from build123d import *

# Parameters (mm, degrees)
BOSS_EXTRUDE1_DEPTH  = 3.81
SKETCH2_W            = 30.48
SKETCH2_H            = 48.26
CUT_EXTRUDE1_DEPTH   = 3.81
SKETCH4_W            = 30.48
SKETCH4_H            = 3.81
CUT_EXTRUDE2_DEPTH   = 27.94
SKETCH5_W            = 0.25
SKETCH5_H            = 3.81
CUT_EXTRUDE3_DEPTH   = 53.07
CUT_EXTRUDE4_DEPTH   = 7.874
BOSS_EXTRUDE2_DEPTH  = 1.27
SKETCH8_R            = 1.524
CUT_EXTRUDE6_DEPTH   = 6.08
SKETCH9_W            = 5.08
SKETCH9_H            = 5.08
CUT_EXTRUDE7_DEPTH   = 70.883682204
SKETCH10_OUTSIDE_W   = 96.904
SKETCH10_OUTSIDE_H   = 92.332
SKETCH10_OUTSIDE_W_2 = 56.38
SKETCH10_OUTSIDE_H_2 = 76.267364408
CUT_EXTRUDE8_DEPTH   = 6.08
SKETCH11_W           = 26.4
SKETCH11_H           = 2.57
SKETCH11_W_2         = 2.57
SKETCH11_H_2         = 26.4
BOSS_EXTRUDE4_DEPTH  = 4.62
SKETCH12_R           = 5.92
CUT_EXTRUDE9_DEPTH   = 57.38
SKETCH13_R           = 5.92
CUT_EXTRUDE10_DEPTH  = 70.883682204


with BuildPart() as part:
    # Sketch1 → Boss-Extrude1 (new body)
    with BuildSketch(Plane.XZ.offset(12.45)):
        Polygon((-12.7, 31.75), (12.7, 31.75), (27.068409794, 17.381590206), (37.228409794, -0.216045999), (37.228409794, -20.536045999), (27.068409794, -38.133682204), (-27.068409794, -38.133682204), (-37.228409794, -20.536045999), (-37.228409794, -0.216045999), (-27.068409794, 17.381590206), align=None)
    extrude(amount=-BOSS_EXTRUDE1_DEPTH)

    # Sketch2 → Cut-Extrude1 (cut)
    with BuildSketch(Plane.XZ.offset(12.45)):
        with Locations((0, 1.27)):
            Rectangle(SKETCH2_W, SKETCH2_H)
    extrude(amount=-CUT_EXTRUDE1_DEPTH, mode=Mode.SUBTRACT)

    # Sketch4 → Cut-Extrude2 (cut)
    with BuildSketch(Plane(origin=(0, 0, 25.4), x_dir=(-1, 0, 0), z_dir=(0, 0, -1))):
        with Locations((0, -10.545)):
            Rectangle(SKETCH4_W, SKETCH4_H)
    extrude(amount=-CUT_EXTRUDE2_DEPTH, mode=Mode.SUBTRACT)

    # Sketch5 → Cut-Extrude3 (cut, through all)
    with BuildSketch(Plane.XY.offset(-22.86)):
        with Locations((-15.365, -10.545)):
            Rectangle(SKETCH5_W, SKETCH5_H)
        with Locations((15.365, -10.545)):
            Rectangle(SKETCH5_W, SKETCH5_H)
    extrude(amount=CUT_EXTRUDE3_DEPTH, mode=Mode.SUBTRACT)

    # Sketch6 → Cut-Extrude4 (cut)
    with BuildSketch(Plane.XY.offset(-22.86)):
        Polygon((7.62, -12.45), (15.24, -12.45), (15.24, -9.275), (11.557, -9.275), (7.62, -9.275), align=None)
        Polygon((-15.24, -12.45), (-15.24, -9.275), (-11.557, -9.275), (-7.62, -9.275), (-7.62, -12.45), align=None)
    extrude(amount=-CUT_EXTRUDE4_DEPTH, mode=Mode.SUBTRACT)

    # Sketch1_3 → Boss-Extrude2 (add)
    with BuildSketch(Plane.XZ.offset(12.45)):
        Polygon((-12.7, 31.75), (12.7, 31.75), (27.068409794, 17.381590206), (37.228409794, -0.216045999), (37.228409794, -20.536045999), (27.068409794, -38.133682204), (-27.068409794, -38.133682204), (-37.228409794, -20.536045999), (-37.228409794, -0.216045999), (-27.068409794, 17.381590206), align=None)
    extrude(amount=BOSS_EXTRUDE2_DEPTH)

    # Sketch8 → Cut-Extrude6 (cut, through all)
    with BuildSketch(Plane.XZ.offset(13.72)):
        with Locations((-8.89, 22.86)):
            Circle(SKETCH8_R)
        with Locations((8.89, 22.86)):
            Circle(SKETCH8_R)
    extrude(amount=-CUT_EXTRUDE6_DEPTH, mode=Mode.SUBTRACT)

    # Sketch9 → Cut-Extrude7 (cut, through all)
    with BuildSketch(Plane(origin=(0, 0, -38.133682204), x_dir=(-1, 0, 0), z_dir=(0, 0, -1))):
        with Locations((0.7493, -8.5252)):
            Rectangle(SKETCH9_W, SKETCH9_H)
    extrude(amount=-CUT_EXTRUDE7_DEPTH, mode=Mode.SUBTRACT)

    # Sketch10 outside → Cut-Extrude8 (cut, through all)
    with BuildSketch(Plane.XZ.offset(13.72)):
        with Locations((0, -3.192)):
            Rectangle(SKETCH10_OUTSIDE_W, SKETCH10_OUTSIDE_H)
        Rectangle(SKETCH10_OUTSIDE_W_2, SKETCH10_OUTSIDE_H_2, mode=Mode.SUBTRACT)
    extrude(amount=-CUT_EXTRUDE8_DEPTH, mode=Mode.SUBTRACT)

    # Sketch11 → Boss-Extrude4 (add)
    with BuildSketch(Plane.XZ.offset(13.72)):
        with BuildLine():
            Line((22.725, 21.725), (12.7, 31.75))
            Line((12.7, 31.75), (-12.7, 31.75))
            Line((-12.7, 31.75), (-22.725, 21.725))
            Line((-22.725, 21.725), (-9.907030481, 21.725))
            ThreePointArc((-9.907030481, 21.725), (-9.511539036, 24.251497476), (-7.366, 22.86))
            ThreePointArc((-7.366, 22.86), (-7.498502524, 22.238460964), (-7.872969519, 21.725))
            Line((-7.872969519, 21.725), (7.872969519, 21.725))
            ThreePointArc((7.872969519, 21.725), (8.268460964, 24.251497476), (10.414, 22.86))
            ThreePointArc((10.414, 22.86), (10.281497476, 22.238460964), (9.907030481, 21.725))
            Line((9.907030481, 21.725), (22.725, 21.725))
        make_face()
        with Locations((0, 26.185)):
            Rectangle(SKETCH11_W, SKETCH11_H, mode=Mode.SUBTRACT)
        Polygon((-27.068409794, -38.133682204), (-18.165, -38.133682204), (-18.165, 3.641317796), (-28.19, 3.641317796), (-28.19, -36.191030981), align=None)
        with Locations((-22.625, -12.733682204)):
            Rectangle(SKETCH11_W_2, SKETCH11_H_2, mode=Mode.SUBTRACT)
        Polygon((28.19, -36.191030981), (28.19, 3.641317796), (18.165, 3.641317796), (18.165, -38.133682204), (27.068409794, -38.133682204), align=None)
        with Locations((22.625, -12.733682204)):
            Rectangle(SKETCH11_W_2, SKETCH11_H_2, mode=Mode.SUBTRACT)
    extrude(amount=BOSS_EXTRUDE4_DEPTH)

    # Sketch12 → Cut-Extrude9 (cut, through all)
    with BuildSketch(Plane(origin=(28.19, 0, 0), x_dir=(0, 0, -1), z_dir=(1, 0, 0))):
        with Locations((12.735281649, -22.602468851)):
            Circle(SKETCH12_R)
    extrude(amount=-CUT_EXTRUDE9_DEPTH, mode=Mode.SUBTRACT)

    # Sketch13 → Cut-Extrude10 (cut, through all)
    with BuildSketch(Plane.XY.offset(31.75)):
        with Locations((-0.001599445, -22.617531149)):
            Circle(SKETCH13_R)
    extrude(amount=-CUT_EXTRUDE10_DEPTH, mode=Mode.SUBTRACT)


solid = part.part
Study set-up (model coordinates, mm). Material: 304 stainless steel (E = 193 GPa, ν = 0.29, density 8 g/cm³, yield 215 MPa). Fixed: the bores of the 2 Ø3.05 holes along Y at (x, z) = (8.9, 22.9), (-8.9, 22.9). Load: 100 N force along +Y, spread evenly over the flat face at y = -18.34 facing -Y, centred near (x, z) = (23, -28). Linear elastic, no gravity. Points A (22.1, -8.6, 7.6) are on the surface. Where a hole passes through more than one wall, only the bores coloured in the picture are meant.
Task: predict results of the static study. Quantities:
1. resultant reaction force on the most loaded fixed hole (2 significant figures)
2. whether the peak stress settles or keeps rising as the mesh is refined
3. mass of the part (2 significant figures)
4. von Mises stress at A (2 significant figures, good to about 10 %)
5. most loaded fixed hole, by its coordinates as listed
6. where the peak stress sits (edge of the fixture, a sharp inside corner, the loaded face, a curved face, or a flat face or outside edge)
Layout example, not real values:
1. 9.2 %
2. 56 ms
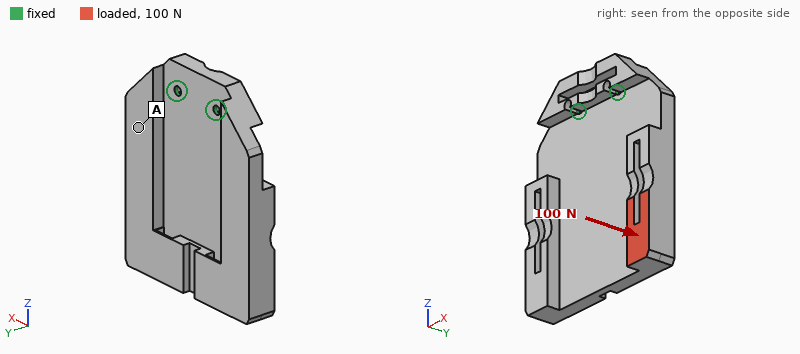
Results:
1. 160 N
2. keeps rising
3. 130 g
4. 32 MPa
5. (8.9, 22.9)
6. edge of the fixture
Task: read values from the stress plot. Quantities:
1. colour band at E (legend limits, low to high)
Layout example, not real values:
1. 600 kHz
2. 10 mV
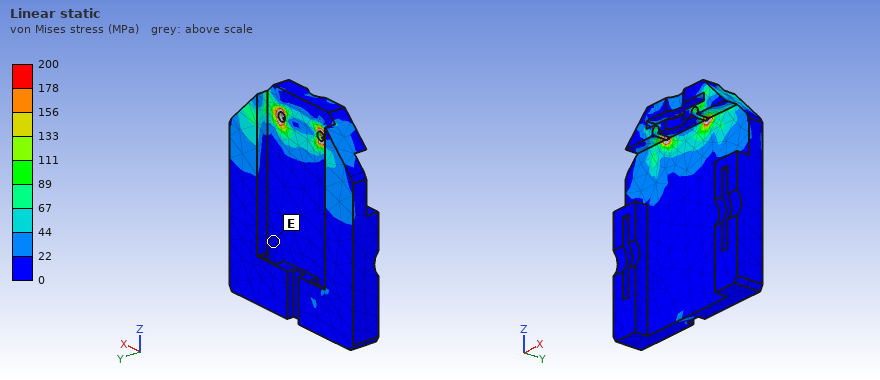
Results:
1. 0 to 22 MPa
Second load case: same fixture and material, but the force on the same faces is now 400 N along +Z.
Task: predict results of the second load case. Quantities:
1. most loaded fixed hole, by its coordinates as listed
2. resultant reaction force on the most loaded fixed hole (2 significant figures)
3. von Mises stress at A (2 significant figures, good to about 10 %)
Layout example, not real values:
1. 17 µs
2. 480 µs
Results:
1. (8.9, 22.9)
2. 670 N
3. 24 MPa
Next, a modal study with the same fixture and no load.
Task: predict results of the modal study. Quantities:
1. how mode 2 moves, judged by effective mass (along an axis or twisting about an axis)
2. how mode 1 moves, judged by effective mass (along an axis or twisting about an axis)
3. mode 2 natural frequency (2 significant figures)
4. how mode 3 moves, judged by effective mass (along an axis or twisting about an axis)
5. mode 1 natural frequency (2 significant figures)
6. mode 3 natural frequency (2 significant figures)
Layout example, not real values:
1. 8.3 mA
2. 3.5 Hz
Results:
1. twisting about Z
2. along Y
3. 1100 Hz
4. along X
5. 370 Hz
6. 2300 Hz
